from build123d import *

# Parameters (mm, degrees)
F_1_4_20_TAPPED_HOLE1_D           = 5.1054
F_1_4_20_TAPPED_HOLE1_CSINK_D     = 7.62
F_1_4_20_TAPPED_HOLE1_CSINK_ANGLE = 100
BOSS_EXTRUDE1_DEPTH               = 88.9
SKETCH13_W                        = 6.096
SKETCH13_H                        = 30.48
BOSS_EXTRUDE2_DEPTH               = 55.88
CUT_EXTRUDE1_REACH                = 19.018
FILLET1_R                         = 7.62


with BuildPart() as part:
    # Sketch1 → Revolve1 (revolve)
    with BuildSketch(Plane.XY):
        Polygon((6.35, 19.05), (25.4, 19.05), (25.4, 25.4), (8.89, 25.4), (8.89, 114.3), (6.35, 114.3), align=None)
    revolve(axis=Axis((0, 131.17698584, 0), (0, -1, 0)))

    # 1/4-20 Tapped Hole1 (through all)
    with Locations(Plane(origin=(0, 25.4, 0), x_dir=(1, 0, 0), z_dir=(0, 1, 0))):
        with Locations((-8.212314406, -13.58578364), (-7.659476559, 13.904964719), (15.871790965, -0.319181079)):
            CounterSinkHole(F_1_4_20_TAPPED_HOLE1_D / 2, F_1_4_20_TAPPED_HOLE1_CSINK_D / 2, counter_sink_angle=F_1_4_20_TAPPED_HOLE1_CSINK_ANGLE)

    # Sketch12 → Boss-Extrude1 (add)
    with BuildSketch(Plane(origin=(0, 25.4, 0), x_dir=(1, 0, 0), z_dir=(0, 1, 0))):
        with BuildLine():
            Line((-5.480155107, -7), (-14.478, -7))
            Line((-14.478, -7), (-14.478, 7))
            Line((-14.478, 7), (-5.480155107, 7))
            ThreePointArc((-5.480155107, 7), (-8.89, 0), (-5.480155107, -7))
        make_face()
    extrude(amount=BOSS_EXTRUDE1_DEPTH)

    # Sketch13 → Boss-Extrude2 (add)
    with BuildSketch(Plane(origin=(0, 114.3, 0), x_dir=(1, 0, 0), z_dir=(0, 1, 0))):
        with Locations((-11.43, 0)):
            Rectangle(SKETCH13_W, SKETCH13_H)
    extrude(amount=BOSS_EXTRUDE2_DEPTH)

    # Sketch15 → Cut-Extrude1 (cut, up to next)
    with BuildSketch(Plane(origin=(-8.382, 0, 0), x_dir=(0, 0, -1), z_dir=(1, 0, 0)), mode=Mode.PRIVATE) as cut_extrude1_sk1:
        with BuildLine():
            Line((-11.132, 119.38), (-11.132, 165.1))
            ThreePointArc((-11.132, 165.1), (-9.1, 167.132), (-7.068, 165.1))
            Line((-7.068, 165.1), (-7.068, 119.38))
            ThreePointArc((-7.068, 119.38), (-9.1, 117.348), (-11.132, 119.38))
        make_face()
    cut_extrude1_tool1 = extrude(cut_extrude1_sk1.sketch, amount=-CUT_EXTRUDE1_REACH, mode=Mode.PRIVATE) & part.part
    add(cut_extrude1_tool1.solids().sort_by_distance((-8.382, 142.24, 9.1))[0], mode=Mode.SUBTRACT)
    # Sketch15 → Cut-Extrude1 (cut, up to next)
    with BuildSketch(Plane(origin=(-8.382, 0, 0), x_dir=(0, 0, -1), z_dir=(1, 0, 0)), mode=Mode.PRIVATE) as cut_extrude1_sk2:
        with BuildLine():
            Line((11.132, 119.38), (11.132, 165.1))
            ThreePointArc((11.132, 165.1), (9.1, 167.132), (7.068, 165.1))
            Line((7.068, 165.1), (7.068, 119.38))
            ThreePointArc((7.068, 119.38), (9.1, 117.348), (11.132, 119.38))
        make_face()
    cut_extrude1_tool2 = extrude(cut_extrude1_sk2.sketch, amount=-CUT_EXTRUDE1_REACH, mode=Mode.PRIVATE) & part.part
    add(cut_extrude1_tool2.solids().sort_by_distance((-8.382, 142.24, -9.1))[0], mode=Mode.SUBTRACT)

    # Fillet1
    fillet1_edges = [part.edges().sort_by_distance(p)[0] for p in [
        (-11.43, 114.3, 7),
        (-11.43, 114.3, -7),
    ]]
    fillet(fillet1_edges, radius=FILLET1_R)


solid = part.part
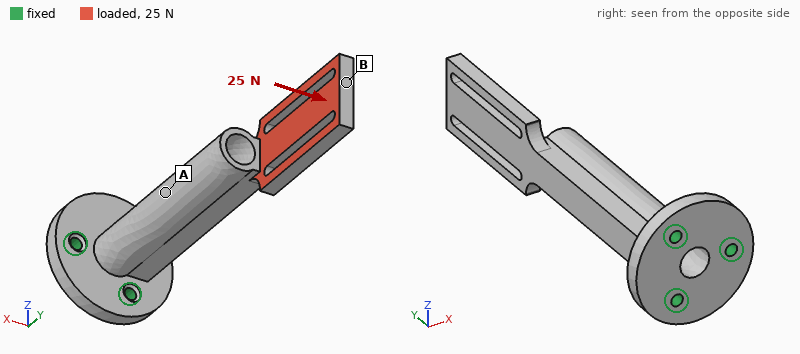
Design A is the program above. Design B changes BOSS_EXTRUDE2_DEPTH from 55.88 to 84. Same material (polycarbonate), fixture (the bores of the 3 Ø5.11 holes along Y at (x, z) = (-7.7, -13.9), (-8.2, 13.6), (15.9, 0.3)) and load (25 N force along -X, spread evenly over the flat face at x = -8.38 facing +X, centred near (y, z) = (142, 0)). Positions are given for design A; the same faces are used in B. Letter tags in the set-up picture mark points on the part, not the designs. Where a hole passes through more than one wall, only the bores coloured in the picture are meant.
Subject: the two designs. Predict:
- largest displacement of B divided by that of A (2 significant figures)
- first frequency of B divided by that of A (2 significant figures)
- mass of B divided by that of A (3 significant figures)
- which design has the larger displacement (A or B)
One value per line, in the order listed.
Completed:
2.2
0.61
1.13
B
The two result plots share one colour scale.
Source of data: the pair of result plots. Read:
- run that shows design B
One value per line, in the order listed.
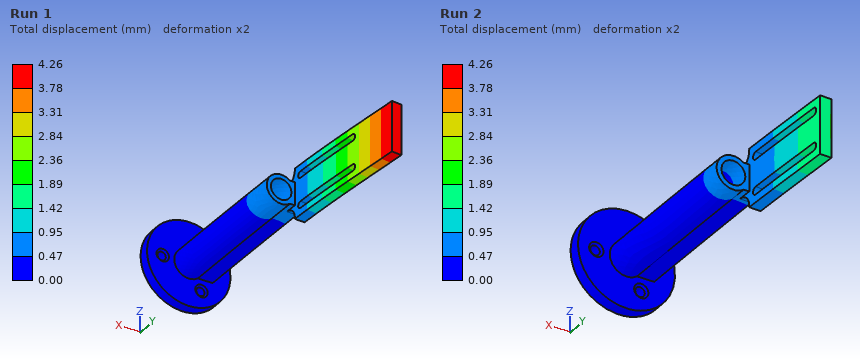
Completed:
Run 1
